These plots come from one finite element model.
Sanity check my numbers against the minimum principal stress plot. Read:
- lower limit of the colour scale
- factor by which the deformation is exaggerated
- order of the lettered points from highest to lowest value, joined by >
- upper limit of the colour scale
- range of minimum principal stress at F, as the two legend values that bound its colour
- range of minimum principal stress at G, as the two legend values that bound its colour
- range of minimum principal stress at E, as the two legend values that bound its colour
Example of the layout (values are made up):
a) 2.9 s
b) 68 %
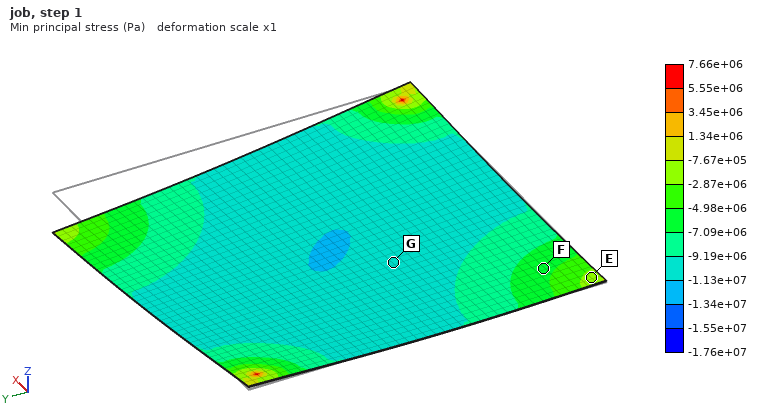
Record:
a) -1.76e+07 Pa
b) 1
c) E > F > G
d) 7.66e+06 Pa
e) -7.09e+06 to -4.98e+06 Pa
f) -1.13e+07 to -9.19e+06 Pa
g) -2.87e+06 to -7.67e+05 Pa
